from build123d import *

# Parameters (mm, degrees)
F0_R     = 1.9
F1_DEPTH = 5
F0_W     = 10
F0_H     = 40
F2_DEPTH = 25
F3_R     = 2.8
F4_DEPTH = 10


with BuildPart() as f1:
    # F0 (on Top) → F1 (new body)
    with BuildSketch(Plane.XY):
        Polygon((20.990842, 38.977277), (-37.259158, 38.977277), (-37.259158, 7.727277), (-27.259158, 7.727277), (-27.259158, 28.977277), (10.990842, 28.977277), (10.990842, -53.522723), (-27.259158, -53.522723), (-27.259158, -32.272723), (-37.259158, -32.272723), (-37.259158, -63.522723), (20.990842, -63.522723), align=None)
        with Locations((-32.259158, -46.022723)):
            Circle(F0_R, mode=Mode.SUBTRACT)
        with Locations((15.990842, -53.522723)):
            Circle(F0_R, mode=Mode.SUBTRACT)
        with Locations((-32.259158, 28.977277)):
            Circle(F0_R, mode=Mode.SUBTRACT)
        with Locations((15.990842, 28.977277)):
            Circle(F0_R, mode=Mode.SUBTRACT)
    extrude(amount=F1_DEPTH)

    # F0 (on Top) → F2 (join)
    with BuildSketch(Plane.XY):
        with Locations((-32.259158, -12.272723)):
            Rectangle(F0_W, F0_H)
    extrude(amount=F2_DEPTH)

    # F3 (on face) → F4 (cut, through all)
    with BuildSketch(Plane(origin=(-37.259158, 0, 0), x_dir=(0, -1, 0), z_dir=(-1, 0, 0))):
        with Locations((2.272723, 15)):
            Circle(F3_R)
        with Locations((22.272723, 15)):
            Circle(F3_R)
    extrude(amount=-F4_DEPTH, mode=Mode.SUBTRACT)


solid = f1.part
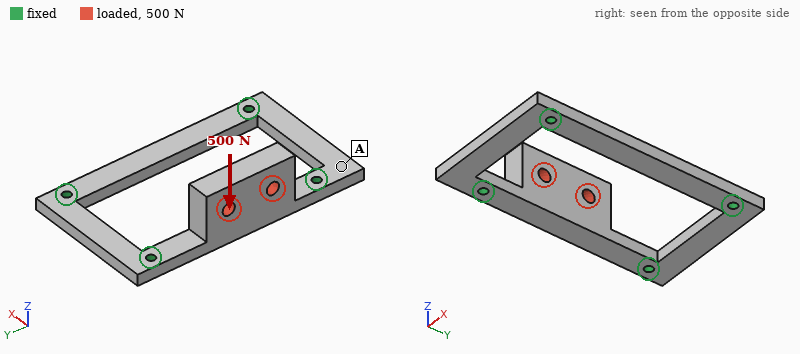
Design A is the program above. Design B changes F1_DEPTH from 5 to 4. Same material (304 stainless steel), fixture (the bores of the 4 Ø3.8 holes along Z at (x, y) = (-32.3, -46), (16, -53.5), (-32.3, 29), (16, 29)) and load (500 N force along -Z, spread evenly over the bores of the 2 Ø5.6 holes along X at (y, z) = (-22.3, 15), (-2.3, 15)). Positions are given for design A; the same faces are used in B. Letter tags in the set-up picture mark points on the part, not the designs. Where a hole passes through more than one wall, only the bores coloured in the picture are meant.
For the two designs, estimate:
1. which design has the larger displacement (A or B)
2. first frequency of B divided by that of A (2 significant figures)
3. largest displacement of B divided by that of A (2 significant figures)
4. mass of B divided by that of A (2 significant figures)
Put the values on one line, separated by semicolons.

B; 0.77; 1.7; 0.89
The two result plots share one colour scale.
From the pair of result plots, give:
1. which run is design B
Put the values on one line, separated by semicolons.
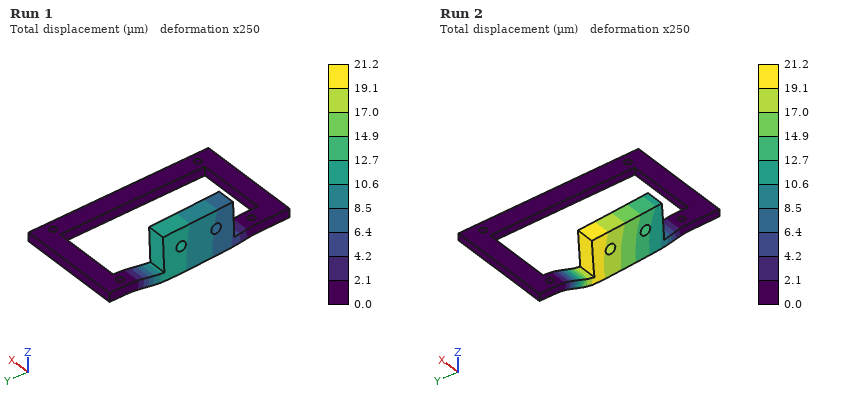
Run 2
